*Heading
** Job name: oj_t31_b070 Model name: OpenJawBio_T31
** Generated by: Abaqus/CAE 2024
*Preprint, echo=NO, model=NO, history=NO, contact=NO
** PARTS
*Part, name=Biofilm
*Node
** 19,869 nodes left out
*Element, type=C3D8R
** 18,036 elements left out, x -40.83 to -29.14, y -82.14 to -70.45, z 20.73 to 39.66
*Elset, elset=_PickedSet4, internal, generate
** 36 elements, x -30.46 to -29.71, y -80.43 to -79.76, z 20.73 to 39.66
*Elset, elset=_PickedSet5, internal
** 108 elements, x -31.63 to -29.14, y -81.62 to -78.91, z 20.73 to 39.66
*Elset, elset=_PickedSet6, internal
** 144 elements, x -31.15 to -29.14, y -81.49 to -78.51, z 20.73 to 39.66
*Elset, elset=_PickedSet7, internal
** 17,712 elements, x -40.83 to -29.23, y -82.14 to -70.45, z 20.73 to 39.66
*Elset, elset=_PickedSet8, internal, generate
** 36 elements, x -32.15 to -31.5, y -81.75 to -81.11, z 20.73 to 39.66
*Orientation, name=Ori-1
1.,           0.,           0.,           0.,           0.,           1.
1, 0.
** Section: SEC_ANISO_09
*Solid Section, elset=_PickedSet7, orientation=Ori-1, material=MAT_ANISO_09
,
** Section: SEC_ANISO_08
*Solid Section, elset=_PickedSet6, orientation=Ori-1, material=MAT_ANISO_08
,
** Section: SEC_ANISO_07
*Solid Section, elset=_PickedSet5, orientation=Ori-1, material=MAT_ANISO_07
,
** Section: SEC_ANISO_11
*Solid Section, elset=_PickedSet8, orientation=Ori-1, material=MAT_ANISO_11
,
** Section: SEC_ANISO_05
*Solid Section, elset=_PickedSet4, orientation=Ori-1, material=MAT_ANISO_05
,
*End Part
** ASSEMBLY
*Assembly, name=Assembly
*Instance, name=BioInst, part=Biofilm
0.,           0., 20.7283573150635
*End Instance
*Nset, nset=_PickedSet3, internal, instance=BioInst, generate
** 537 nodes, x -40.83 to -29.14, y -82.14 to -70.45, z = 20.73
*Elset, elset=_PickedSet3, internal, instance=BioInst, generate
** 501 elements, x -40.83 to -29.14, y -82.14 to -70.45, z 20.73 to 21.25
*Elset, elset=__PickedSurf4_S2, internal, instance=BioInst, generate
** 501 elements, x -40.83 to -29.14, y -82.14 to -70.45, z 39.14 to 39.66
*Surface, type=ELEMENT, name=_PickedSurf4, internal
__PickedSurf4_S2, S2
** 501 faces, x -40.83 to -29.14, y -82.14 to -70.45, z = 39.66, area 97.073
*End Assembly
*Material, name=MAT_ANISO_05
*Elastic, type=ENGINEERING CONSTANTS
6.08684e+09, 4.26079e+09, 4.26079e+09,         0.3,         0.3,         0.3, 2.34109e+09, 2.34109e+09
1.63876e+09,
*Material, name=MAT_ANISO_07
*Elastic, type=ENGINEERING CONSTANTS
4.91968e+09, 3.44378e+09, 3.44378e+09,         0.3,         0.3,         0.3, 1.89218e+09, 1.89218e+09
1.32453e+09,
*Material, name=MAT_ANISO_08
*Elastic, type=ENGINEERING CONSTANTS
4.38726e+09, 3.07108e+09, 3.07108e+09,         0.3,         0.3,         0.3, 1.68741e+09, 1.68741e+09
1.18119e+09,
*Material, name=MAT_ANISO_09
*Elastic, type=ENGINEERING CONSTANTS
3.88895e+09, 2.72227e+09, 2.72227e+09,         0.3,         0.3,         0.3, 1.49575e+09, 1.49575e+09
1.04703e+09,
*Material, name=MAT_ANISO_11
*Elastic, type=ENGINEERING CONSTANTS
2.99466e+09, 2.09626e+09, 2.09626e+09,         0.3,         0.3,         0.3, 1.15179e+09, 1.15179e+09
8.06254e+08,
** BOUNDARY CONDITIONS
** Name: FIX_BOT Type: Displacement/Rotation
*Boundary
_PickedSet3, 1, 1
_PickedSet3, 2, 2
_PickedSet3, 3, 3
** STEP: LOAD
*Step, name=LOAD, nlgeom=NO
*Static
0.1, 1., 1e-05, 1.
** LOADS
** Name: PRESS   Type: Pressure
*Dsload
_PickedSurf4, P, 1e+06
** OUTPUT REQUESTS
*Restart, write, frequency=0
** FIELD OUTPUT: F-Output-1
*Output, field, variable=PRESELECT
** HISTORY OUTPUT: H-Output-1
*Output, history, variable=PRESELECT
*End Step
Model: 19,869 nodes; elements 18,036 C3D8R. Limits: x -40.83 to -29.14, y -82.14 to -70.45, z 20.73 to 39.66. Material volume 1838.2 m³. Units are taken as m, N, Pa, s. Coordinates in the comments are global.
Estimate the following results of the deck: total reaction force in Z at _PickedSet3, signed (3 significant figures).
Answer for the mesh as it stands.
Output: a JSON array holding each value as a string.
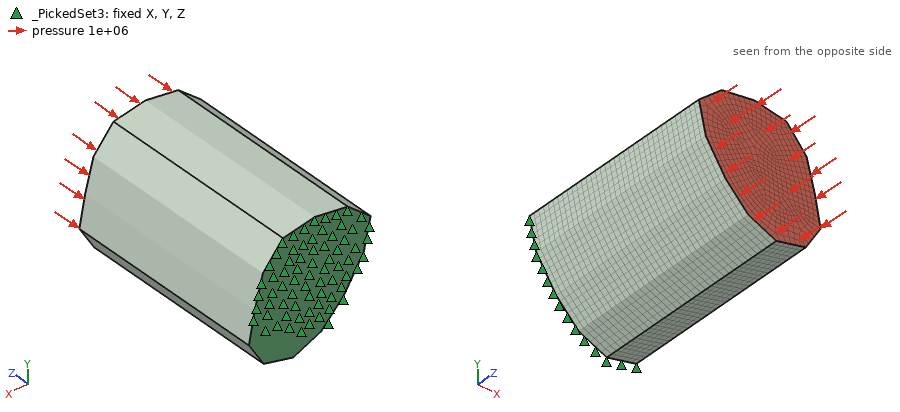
["9.71e+07 N"]
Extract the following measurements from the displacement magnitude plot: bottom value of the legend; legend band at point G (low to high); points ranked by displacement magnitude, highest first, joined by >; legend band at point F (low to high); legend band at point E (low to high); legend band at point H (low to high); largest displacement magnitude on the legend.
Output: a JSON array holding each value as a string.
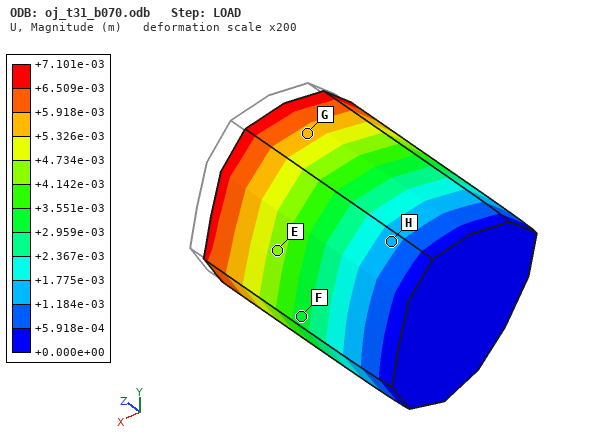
["+0.000e+00 m", "+5.326e-03 to +5.918e-03 m", "G > E > F > H", "+2.959e-03 to +3.551e-03 m", "+4.142e-03 to +4.734e-03 m", "+1.184e-03 to +1.775e-03 m", "+7.101e-03 m"]
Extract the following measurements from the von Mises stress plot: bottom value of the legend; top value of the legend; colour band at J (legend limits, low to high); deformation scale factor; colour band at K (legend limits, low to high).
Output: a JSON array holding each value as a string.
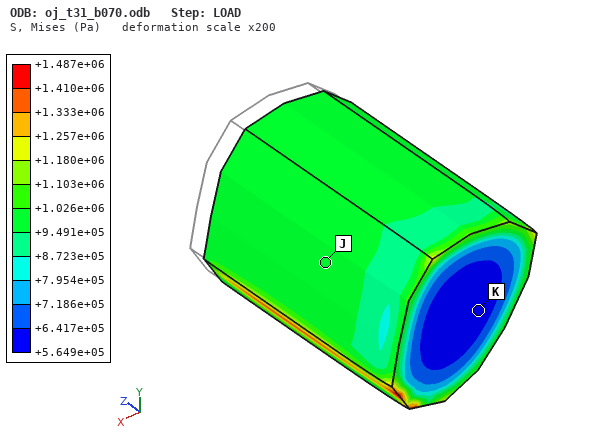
["+5.649e+05 Pa", "+1.487e+06 Pa", "+9.491e+05 to +1.026e+06 Pa", "200", "+5.649e+05 to +6.417e+05 Pa"]
